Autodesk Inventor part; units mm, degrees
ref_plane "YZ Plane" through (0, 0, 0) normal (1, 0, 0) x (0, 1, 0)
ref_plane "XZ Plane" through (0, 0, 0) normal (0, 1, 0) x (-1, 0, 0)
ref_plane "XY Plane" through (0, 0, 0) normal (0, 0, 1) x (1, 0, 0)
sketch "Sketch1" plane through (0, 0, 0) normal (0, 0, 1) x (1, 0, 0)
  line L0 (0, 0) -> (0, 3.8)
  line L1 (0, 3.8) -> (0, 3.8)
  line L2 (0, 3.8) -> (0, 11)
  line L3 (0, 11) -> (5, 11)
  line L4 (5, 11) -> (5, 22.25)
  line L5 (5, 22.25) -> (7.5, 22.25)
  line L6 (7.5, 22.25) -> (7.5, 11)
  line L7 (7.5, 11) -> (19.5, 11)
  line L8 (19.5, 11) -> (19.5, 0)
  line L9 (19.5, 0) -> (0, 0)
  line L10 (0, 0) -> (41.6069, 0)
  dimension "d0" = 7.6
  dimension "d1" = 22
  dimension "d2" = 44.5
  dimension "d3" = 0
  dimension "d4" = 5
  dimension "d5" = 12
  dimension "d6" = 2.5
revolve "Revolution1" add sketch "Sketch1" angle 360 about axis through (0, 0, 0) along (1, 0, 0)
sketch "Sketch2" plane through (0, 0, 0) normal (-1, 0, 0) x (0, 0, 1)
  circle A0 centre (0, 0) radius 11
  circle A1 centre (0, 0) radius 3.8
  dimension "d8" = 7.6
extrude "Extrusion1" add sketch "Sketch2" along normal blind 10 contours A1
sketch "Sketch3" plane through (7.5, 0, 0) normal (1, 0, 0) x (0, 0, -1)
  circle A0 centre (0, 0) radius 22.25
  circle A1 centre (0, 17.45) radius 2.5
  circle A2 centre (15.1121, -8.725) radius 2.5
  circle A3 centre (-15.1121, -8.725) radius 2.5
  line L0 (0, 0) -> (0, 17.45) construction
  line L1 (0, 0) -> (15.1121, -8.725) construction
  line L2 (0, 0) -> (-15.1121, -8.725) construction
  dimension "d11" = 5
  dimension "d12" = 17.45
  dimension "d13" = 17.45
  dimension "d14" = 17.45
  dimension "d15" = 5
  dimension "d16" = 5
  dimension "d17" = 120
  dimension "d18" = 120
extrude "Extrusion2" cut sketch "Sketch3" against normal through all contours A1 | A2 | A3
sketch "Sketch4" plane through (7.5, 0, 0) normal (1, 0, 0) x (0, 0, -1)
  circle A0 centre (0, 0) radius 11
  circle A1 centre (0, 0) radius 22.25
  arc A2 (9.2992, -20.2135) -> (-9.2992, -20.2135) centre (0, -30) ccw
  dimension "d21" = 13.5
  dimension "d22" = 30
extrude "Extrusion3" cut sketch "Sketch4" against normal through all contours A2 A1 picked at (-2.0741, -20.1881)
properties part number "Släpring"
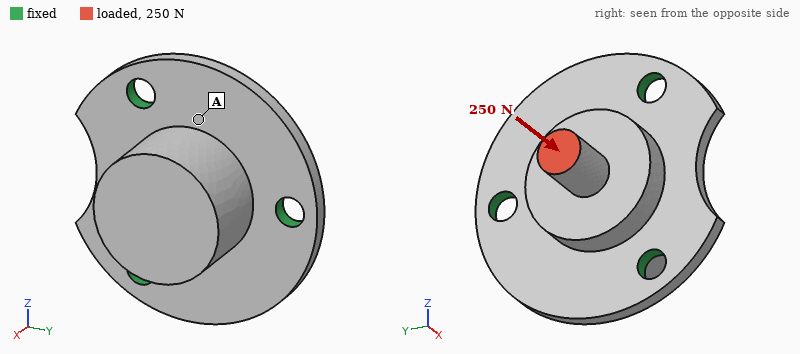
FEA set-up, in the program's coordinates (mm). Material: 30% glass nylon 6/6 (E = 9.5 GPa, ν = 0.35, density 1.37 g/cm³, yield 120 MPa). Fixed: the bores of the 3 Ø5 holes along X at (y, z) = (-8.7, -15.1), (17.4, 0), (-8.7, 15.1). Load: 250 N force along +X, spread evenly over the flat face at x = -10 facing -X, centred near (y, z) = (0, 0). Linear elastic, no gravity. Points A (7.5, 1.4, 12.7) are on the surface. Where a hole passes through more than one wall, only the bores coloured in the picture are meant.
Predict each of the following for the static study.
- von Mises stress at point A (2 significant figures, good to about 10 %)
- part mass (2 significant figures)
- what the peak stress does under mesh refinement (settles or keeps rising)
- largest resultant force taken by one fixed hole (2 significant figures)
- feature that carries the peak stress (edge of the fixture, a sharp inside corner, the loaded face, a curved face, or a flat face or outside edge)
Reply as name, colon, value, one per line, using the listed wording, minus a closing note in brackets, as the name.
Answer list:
von Mises stress at point A: 3.1 MPa
part mass: 14 g
what the peak stress does under mesh refinement: keeps rising
largest resultant force taken by one fixed hole: 84 N
feature that carries the peak stress: edge of the fixture
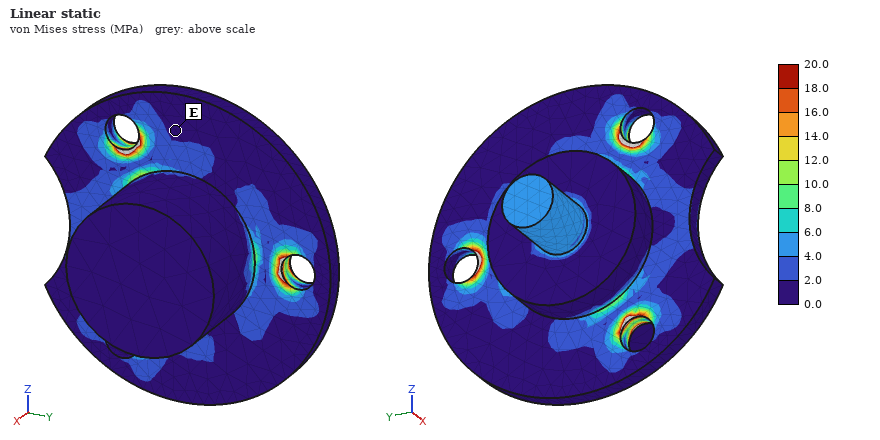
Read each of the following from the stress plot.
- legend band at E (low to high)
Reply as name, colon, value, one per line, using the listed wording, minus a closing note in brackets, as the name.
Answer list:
legend band at E: 0.0 to 2.0 MPa
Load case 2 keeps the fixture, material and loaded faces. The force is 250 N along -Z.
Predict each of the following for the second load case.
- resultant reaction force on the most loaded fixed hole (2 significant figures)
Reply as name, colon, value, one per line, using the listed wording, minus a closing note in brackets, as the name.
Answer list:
resultant reaction force on the most loaded fixed hole: 180 N
